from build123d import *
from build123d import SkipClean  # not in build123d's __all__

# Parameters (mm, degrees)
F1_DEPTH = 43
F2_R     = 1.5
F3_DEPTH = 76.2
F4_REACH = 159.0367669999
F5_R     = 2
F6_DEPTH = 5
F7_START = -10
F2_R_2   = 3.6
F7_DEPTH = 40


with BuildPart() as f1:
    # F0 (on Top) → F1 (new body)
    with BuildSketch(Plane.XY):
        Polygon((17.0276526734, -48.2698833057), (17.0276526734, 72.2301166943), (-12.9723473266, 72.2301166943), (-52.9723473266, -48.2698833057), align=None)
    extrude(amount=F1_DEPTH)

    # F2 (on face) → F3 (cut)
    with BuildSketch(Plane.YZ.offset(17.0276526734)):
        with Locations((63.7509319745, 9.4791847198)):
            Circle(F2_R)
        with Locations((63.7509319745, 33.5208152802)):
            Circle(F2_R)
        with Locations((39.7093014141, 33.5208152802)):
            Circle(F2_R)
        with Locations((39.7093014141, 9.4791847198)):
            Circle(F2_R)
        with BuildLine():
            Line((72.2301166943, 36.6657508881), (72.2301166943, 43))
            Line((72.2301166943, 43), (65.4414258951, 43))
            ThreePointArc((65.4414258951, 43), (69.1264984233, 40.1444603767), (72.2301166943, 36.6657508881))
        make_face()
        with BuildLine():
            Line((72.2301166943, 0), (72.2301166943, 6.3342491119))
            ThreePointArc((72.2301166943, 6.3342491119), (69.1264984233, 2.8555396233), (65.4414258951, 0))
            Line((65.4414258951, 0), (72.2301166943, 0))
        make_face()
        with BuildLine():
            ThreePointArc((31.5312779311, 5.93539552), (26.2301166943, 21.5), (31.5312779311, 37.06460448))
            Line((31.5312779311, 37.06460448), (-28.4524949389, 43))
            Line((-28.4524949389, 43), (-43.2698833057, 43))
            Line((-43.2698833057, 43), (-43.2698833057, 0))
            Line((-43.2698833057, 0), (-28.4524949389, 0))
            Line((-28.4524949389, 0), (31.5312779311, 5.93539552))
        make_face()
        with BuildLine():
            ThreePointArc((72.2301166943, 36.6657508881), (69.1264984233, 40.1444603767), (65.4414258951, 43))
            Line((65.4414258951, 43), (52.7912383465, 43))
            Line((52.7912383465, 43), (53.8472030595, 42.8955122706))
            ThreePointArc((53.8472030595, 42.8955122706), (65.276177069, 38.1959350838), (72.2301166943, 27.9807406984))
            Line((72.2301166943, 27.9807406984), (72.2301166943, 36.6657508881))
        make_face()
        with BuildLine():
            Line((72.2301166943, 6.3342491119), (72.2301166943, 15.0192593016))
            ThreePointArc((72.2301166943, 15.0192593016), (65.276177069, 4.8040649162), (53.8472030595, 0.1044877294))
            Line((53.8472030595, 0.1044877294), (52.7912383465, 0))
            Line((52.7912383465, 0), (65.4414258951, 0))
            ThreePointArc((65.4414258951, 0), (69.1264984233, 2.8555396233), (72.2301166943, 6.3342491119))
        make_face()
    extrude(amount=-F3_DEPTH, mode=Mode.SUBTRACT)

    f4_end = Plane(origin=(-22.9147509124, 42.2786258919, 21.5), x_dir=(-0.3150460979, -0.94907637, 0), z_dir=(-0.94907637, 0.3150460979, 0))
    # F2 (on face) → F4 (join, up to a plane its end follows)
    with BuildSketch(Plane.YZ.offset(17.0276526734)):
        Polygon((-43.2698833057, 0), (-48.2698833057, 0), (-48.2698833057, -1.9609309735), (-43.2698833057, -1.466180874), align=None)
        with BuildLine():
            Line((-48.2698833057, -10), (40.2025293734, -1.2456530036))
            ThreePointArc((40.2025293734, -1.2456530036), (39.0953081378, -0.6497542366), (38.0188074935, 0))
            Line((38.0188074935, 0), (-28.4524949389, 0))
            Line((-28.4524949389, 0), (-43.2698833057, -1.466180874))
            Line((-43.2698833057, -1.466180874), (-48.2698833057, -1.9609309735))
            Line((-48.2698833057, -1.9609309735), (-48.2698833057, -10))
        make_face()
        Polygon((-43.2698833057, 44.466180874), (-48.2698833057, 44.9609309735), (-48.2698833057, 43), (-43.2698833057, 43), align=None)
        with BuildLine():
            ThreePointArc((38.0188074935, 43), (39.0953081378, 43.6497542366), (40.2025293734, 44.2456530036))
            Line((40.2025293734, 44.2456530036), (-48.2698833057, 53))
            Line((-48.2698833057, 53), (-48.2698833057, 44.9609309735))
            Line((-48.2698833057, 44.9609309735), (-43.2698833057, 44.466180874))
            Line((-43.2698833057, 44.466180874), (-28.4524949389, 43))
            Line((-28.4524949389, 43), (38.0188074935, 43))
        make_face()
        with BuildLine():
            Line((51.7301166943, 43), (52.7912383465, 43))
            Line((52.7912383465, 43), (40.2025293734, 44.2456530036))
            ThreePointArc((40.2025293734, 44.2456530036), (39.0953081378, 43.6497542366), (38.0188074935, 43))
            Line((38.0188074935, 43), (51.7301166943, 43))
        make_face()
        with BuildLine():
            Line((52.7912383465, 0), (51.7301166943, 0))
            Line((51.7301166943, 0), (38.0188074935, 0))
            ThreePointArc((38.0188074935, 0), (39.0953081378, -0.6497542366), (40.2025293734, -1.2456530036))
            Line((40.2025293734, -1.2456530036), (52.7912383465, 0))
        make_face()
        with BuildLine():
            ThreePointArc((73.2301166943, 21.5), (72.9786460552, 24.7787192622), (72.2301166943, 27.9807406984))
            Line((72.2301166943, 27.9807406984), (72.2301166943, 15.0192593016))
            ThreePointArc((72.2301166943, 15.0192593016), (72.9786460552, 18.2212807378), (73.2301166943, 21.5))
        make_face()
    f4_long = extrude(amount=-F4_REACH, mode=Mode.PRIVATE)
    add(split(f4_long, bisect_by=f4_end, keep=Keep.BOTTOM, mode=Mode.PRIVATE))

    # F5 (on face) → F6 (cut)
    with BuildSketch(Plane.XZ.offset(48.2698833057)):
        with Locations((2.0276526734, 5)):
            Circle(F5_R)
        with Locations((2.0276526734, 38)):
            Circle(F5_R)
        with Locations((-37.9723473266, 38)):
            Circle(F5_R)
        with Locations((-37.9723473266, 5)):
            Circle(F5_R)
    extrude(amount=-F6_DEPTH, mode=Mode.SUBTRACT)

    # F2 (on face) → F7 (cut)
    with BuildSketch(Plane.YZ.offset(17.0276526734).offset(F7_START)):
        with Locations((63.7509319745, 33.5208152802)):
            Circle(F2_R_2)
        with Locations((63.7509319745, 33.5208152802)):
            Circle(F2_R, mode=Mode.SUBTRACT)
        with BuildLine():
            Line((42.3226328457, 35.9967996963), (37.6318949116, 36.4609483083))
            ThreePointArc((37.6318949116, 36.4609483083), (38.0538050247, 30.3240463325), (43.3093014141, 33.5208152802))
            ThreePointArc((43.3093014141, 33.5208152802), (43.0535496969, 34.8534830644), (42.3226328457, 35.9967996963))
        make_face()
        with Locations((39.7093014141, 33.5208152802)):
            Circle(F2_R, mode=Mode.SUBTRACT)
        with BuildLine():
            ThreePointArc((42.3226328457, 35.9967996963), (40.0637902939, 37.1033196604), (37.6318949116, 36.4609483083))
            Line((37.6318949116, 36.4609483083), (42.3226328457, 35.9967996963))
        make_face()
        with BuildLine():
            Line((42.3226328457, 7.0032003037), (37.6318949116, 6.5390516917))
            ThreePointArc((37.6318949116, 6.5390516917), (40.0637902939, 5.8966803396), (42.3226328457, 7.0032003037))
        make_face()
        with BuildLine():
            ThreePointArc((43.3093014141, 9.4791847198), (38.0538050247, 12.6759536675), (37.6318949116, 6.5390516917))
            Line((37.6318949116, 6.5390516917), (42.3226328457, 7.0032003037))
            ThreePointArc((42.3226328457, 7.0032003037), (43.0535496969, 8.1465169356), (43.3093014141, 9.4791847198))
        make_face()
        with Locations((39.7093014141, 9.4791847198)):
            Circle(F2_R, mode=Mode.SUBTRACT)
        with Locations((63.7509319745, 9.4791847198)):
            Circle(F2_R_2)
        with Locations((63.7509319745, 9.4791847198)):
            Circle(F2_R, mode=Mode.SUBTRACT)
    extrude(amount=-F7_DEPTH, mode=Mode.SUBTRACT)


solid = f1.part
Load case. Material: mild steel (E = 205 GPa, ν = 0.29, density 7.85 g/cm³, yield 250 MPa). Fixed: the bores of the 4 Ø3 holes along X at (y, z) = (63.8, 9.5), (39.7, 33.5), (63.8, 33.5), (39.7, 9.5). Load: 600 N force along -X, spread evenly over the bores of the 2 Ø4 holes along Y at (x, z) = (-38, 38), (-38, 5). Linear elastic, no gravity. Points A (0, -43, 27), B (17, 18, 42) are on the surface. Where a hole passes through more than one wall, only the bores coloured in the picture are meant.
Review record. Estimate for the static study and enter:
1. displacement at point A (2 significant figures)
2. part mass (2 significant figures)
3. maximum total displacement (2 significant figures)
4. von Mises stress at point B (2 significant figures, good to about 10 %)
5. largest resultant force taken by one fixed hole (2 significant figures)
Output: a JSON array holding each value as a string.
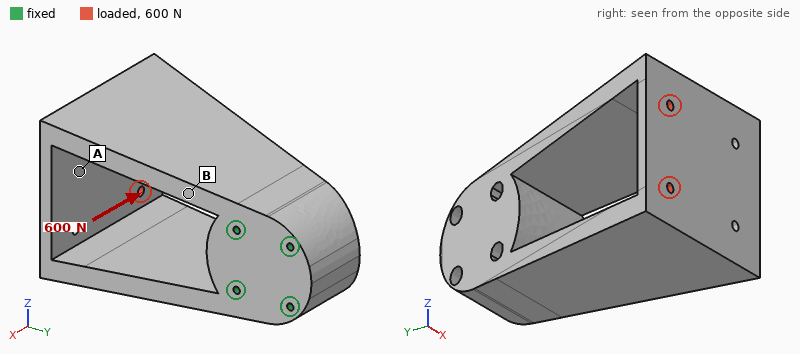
["12 µm", "1.2 kg", "15 µm", "6.6 MPa", "1.2 kN"]
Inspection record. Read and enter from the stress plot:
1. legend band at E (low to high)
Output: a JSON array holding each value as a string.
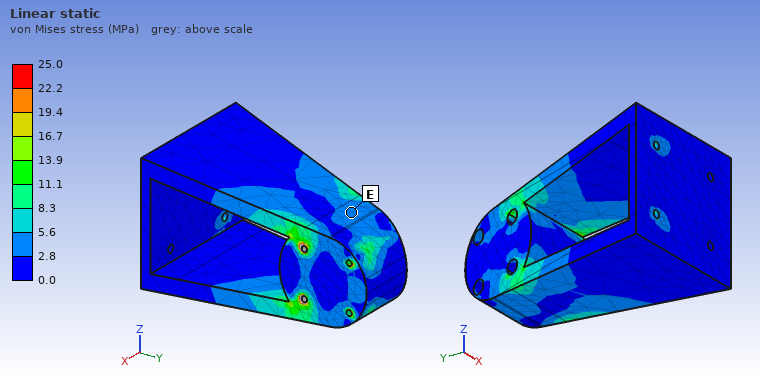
["2.8 to 5.6 MPa"]
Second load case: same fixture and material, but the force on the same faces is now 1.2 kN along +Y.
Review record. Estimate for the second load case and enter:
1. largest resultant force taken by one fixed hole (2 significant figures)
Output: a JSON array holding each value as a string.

["1.1 kN"]
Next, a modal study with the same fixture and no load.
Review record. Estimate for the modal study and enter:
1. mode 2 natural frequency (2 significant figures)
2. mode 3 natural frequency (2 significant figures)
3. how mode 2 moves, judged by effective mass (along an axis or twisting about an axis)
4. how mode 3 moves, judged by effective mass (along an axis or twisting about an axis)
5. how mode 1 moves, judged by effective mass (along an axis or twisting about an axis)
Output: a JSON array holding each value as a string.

["1700 Hz", "2300 Hz", "along X", "twisting about Y", "along Z"]
